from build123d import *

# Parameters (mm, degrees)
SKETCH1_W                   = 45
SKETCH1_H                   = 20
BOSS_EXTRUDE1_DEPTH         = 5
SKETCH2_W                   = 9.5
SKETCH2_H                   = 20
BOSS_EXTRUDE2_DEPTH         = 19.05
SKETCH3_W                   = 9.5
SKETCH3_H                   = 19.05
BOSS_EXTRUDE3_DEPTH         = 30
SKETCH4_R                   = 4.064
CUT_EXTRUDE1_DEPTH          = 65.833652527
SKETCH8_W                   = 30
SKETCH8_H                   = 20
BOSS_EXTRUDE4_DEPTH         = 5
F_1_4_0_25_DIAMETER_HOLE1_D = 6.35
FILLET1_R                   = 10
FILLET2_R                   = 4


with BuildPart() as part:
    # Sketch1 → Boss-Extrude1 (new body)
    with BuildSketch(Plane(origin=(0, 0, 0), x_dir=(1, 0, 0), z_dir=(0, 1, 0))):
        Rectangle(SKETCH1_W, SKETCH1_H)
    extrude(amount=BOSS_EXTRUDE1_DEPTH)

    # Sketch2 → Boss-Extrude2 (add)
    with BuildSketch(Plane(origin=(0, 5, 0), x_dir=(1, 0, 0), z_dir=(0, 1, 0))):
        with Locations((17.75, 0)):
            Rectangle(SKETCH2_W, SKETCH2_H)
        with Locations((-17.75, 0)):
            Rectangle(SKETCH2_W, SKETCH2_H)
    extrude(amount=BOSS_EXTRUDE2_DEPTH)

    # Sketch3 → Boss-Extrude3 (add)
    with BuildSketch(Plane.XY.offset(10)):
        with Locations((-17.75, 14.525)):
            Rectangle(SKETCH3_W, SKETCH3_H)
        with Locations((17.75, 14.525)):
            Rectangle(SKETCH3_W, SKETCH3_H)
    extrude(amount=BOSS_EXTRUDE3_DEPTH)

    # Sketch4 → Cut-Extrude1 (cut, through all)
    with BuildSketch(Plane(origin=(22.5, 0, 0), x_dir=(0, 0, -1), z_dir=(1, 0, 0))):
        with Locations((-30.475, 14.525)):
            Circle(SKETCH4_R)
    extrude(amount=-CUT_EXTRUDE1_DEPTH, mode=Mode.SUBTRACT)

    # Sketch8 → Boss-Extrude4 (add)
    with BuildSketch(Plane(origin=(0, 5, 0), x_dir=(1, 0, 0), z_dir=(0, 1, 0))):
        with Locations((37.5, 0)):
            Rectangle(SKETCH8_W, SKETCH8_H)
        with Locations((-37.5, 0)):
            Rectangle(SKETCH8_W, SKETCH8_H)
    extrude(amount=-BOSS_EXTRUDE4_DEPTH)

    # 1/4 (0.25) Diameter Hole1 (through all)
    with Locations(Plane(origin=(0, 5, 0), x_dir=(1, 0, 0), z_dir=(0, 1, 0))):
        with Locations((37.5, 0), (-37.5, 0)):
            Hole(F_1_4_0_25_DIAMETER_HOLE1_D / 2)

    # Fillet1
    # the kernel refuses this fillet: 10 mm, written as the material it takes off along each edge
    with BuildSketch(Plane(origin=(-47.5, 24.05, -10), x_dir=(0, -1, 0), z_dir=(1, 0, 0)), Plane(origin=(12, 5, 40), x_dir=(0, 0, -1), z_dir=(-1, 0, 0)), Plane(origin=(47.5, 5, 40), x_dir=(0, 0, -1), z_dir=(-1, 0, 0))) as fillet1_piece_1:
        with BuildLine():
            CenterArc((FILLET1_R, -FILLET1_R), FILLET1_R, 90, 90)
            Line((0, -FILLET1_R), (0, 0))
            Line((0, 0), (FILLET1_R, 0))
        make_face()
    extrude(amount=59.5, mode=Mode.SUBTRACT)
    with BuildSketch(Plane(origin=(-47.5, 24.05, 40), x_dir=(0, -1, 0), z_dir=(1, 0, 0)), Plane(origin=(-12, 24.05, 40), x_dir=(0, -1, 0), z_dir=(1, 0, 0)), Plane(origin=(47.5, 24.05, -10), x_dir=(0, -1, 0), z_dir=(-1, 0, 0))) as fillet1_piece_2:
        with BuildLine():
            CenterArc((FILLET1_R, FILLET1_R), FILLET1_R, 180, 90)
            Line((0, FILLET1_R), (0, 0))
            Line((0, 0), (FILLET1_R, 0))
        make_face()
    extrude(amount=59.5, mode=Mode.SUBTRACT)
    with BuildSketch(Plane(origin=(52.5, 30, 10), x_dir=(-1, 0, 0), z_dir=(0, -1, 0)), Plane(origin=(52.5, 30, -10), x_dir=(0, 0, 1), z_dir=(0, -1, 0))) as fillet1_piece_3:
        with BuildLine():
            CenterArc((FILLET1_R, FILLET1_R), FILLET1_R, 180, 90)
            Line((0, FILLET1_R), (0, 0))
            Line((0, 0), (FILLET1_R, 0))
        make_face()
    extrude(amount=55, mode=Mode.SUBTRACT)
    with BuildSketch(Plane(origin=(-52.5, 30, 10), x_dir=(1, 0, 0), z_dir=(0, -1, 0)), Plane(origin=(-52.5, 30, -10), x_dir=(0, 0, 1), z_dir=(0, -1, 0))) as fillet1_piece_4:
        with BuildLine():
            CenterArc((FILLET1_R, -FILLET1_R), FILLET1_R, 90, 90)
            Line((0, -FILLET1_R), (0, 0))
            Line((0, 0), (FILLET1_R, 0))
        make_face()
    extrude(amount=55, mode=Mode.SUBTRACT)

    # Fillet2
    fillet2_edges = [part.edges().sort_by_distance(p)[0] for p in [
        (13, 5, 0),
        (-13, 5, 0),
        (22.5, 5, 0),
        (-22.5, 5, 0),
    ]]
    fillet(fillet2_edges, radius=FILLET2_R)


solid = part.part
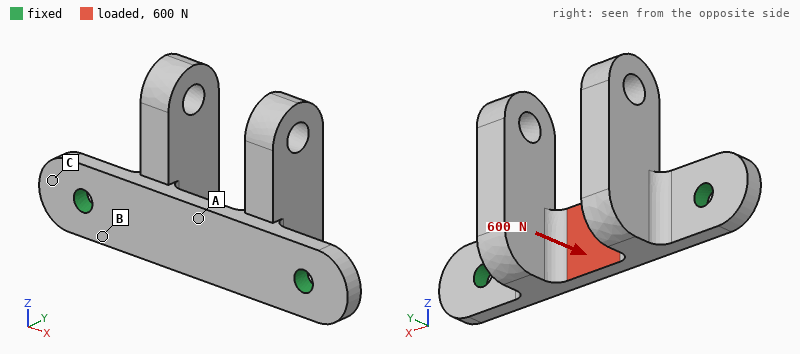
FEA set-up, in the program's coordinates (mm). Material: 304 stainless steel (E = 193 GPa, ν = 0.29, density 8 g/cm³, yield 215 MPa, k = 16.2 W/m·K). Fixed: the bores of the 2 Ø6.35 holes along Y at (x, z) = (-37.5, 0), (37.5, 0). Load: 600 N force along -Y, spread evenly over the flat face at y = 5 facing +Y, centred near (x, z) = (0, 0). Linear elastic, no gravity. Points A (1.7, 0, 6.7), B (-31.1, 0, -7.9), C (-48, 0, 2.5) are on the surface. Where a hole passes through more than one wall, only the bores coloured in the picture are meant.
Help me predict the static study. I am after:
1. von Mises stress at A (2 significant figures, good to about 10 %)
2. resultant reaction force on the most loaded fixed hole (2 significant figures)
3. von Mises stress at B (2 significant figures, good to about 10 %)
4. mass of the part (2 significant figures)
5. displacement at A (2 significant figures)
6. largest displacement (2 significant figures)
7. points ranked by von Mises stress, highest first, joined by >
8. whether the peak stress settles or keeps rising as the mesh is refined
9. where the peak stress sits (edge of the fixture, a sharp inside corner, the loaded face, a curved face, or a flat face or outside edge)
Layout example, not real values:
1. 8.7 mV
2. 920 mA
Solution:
1. 49 MPa
2. 300 N
3. 36 MPa
4. 210 g
5. 28 µm
6. 30 µm
7. A > B > C
8. keeps rising
9. edge of the fixture
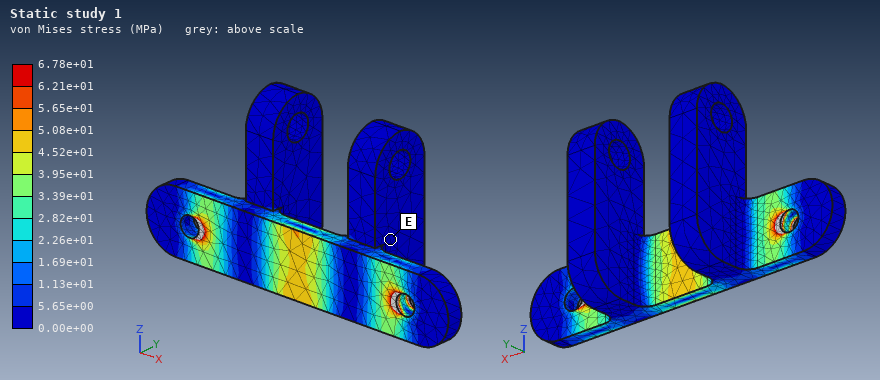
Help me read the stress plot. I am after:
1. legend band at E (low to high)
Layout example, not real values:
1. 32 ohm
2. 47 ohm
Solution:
1. 0.00e+00 to 5.65e+00 MPa
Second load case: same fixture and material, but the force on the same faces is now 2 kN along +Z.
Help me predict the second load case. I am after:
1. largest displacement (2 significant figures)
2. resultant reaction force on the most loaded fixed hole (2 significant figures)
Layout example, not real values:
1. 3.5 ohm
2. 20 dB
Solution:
1. 28 µm
2. 1.0 kN
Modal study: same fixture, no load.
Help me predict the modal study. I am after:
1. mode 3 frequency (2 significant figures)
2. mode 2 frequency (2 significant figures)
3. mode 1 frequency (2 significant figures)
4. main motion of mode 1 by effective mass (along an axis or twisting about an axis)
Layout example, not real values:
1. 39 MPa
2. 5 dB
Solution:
1. 2700 Hz
2. 2600 Hz
3. 1800 Hz
4. along Y
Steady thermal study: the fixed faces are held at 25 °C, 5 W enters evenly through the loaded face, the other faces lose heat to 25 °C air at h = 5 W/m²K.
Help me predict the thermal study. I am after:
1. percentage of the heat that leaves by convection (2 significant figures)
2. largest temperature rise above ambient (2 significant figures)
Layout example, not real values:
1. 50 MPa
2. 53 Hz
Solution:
1. 17 %
2. 39 K
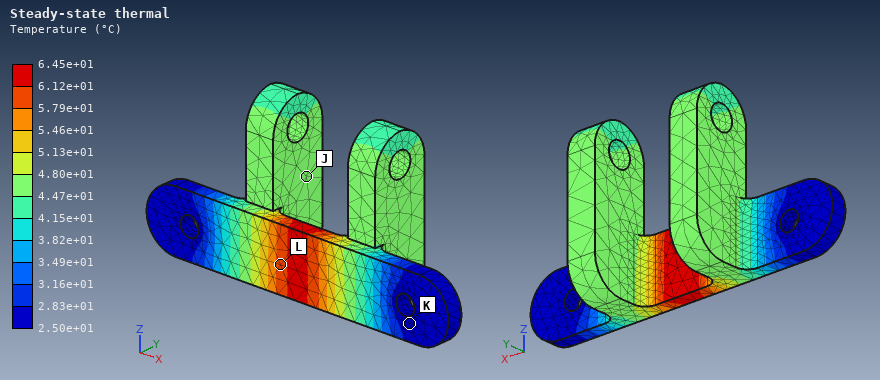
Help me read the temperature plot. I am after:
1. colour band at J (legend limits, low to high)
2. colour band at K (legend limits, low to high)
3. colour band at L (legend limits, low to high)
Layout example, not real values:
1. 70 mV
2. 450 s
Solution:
1. 4.47e+01 to 4.80e+01 °C
2. 2.50e+01 to 2.83e+01 °C
3. 5.79e+01 to 6.12e+01 °C
